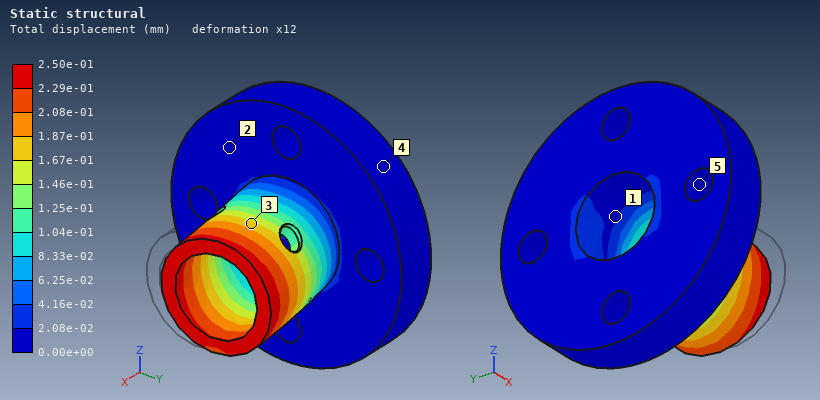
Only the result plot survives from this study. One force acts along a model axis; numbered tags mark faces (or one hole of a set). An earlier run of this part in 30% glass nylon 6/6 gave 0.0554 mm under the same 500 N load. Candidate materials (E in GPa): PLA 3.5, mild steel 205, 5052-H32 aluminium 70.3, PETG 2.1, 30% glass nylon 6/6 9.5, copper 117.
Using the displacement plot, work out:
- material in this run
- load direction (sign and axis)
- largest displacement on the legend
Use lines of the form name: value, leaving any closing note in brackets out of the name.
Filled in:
material in this run: PETG
load direction: +Y
largest displacement on the legend: 2.50e-01 mm
